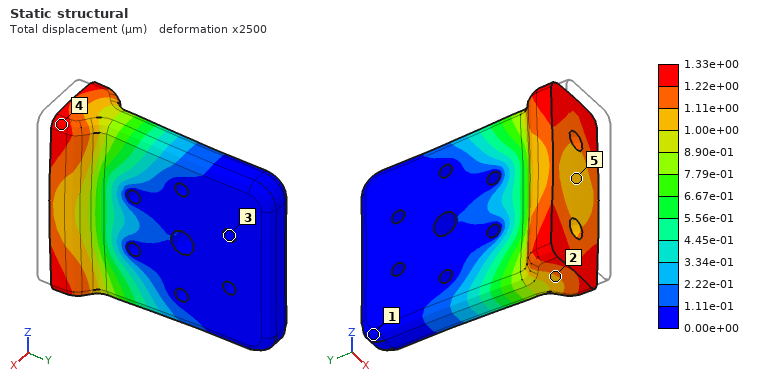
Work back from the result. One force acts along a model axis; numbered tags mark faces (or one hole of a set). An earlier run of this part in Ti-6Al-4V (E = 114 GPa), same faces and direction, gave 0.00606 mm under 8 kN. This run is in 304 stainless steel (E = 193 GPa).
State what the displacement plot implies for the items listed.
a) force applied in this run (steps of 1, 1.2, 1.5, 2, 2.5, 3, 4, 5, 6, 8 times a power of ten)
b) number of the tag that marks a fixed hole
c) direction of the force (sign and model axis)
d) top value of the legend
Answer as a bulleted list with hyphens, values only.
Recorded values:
- 3 kN
- 3
- +Y
- 1.33e+00 µm
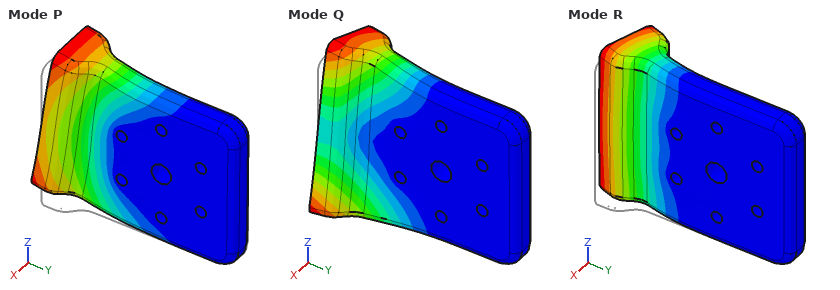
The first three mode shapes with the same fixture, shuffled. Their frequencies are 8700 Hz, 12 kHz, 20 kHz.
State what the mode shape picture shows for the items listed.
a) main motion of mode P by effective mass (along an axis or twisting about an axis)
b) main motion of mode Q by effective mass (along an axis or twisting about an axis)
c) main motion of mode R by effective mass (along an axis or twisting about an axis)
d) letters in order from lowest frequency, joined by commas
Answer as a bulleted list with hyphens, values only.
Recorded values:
- along Z
- twisting about Y
- along X
- R, Q, P
